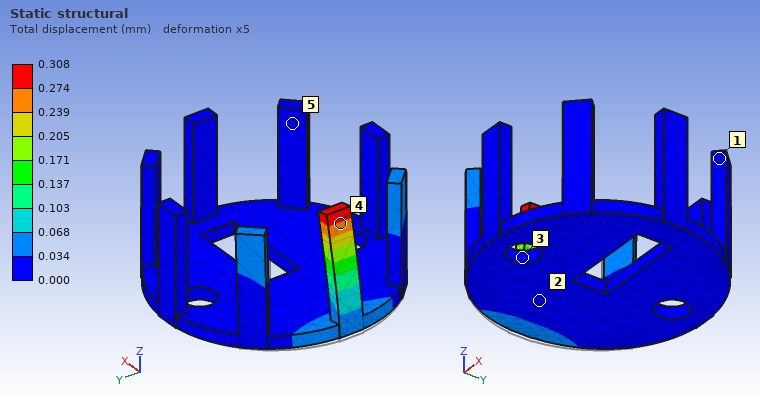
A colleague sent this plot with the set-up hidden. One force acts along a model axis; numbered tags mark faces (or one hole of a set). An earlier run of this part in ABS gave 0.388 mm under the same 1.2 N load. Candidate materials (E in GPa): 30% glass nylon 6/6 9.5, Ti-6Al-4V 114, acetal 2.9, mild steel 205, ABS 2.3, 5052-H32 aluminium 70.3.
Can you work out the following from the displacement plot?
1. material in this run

acetal
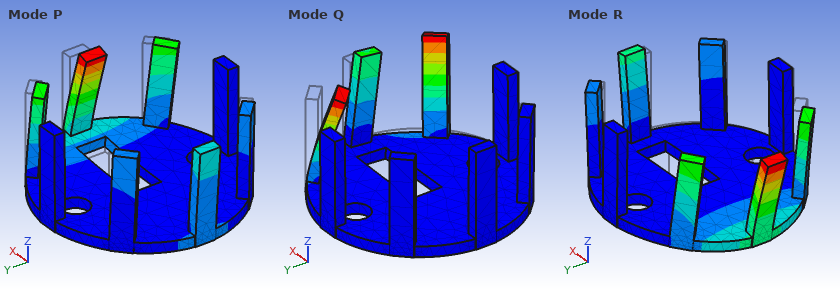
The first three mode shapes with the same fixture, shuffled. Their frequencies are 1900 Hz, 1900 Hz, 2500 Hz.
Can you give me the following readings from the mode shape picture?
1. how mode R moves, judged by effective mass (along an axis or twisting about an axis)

along Z
